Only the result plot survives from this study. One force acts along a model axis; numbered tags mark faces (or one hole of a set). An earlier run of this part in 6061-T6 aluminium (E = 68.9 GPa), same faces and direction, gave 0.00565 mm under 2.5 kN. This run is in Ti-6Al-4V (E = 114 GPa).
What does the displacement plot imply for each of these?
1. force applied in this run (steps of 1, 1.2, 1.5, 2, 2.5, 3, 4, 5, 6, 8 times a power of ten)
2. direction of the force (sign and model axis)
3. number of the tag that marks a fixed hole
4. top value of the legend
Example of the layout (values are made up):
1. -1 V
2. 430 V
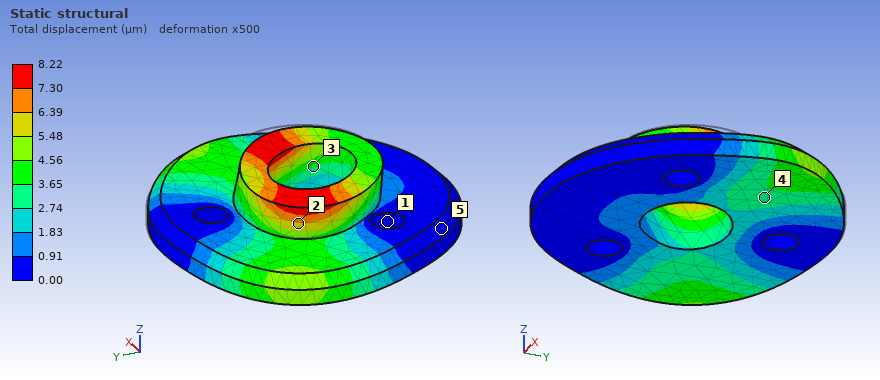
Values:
1. 6 kN
2. -X
3. 1
4. 8.22 µm
